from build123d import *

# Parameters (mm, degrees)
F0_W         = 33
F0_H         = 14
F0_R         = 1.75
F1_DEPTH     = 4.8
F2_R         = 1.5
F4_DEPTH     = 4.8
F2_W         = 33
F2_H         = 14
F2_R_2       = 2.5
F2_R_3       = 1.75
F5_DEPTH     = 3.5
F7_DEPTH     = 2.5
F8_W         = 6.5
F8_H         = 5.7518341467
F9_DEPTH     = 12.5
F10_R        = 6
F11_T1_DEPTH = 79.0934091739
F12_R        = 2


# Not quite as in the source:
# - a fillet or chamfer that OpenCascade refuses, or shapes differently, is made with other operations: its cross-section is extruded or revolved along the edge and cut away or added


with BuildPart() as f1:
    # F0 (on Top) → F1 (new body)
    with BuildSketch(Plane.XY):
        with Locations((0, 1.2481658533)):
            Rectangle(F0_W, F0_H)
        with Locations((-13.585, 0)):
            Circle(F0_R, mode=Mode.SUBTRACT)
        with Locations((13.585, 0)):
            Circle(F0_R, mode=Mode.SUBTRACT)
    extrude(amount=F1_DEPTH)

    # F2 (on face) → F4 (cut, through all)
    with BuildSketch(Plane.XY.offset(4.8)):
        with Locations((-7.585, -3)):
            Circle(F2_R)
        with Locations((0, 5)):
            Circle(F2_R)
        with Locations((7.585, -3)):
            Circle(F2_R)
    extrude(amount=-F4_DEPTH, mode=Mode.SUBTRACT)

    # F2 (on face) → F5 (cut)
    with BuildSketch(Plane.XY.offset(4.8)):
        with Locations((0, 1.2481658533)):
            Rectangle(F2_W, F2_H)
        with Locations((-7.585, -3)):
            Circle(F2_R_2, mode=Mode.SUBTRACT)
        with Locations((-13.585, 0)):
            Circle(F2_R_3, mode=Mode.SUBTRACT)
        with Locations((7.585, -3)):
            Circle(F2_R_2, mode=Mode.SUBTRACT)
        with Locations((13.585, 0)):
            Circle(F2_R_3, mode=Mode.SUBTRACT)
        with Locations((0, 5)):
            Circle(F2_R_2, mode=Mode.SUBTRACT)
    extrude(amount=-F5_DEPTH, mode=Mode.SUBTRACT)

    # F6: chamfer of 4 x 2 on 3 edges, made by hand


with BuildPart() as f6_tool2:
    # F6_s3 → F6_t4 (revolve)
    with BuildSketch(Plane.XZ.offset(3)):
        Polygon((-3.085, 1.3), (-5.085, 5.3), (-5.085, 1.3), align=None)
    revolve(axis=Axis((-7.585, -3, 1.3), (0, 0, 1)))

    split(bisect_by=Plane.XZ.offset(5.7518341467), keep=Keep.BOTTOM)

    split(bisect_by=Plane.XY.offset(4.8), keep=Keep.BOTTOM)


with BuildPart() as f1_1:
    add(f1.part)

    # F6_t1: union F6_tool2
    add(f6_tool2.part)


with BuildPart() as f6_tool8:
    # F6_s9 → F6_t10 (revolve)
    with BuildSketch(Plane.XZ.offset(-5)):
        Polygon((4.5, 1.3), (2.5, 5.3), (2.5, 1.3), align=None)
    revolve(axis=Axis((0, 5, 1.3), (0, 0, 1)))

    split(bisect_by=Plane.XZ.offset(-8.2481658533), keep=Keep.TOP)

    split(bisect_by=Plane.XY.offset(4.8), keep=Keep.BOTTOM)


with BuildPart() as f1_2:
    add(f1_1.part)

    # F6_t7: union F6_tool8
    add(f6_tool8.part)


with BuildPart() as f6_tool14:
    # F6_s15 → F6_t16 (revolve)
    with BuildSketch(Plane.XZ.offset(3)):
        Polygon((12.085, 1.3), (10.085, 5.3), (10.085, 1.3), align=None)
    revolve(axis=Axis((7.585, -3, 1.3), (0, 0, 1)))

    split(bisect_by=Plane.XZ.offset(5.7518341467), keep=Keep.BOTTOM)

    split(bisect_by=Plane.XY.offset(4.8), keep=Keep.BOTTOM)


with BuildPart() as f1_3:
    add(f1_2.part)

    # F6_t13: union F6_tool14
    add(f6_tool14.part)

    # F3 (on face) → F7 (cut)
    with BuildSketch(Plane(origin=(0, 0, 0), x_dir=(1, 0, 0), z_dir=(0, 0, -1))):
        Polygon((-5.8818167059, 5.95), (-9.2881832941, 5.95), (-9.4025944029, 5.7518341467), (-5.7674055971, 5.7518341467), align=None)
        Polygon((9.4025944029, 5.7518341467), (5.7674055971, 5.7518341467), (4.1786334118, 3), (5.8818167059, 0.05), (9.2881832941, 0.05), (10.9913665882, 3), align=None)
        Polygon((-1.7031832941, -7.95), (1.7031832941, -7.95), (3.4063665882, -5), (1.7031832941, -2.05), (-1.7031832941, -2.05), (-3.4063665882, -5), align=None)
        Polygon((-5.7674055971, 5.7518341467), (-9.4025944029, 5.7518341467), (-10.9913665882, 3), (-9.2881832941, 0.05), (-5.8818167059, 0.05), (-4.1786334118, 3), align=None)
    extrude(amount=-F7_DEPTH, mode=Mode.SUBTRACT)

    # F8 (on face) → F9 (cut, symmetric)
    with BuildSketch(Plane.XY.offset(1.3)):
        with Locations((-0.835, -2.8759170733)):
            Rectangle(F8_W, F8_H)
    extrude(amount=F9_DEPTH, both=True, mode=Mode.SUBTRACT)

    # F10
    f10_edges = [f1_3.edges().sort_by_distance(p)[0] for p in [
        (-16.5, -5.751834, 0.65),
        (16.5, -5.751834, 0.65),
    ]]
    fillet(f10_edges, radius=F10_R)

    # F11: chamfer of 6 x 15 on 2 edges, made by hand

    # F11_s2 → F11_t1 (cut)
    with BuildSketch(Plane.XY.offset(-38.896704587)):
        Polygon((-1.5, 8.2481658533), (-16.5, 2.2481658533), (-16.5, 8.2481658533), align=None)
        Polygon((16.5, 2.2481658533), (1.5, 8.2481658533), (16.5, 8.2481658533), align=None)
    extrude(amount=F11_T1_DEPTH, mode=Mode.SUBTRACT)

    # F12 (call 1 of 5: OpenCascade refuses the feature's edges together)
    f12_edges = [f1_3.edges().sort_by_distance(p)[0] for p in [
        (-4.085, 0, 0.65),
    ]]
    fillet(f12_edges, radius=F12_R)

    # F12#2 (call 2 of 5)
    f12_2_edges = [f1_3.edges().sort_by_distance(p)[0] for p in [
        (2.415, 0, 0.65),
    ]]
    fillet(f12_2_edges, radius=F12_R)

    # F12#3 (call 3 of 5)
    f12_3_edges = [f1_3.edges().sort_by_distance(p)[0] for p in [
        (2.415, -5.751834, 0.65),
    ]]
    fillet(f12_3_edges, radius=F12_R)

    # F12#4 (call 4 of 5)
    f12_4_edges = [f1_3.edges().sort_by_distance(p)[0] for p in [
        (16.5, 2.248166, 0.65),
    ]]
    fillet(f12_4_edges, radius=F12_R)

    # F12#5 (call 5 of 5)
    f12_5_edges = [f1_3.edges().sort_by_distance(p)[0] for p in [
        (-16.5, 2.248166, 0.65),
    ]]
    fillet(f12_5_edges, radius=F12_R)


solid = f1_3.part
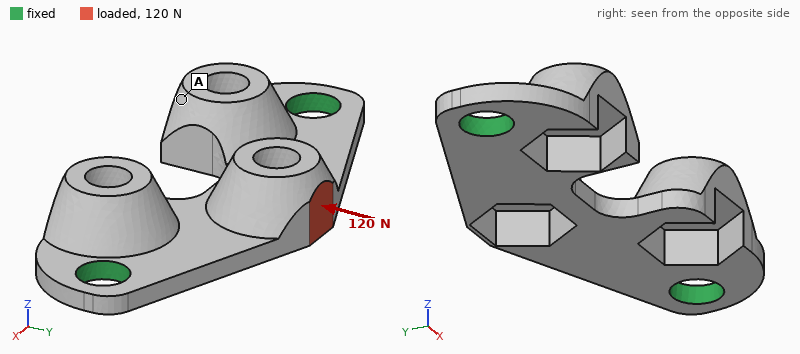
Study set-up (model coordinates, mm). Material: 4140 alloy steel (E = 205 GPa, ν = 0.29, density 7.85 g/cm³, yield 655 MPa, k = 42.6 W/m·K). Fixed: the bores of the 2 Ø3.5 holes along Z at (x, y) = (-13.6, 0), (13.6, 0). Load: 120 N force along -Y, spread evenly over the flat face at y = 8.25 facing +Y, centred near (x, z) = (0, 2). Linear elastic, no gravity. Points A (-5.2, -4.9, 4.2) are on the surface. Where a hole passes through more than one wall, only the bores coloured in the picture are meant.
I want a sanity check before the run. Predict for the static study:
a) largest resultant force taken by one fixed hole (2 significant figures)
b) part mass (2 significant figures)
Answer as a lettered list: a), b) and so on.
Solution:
a) 72 N
b) 4.1 g
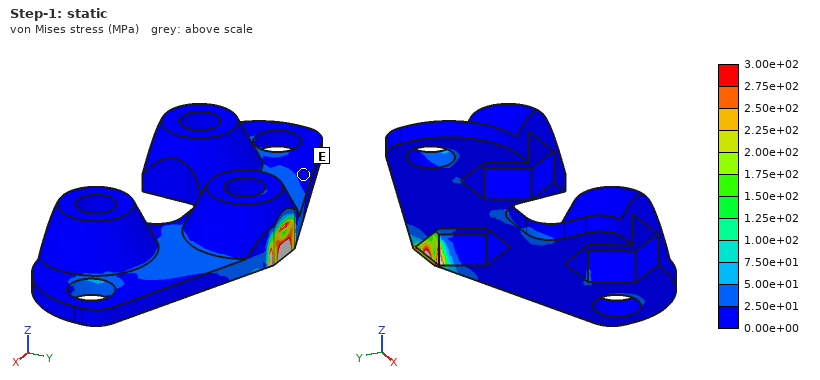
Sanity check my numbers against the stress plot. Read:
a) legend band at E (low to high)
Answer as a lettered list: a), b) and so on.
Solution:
a) 0.00e+00 to 2.50e+01 MPa
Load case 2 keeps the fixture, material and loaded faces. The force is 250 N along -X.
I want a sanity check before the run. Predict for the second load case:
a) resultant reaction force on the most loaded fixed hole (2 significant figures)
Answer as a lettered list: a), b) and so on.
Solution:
a) 150 N
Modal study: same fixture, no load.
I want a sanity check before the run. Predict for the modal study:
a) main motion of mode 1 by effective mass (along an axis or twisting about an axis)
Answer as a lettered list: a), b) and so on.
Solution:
a) along Z
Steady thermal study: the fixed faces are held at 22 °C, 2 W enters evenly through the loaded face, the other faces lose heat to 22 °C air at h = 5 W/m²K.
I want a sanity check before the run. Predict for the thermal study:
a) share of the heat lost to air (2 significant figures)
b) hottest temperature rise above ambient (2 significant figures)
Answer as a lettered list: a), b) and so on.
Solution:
a) 3.1 %
b) 60 K
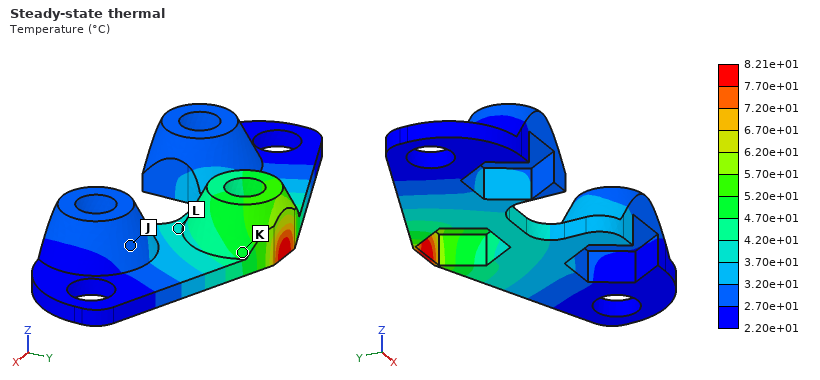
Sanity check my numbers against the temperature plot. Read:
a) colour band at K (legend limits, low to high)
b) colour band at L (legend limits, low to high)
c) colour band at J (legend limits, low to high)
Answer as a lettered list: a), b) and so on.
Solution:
a) 4.70e+01 to 5.20e+01 °C
b) 3.70e+01 to 4.20e+01 °C
c) 2.70e+01 to 3.20e+01 °C
